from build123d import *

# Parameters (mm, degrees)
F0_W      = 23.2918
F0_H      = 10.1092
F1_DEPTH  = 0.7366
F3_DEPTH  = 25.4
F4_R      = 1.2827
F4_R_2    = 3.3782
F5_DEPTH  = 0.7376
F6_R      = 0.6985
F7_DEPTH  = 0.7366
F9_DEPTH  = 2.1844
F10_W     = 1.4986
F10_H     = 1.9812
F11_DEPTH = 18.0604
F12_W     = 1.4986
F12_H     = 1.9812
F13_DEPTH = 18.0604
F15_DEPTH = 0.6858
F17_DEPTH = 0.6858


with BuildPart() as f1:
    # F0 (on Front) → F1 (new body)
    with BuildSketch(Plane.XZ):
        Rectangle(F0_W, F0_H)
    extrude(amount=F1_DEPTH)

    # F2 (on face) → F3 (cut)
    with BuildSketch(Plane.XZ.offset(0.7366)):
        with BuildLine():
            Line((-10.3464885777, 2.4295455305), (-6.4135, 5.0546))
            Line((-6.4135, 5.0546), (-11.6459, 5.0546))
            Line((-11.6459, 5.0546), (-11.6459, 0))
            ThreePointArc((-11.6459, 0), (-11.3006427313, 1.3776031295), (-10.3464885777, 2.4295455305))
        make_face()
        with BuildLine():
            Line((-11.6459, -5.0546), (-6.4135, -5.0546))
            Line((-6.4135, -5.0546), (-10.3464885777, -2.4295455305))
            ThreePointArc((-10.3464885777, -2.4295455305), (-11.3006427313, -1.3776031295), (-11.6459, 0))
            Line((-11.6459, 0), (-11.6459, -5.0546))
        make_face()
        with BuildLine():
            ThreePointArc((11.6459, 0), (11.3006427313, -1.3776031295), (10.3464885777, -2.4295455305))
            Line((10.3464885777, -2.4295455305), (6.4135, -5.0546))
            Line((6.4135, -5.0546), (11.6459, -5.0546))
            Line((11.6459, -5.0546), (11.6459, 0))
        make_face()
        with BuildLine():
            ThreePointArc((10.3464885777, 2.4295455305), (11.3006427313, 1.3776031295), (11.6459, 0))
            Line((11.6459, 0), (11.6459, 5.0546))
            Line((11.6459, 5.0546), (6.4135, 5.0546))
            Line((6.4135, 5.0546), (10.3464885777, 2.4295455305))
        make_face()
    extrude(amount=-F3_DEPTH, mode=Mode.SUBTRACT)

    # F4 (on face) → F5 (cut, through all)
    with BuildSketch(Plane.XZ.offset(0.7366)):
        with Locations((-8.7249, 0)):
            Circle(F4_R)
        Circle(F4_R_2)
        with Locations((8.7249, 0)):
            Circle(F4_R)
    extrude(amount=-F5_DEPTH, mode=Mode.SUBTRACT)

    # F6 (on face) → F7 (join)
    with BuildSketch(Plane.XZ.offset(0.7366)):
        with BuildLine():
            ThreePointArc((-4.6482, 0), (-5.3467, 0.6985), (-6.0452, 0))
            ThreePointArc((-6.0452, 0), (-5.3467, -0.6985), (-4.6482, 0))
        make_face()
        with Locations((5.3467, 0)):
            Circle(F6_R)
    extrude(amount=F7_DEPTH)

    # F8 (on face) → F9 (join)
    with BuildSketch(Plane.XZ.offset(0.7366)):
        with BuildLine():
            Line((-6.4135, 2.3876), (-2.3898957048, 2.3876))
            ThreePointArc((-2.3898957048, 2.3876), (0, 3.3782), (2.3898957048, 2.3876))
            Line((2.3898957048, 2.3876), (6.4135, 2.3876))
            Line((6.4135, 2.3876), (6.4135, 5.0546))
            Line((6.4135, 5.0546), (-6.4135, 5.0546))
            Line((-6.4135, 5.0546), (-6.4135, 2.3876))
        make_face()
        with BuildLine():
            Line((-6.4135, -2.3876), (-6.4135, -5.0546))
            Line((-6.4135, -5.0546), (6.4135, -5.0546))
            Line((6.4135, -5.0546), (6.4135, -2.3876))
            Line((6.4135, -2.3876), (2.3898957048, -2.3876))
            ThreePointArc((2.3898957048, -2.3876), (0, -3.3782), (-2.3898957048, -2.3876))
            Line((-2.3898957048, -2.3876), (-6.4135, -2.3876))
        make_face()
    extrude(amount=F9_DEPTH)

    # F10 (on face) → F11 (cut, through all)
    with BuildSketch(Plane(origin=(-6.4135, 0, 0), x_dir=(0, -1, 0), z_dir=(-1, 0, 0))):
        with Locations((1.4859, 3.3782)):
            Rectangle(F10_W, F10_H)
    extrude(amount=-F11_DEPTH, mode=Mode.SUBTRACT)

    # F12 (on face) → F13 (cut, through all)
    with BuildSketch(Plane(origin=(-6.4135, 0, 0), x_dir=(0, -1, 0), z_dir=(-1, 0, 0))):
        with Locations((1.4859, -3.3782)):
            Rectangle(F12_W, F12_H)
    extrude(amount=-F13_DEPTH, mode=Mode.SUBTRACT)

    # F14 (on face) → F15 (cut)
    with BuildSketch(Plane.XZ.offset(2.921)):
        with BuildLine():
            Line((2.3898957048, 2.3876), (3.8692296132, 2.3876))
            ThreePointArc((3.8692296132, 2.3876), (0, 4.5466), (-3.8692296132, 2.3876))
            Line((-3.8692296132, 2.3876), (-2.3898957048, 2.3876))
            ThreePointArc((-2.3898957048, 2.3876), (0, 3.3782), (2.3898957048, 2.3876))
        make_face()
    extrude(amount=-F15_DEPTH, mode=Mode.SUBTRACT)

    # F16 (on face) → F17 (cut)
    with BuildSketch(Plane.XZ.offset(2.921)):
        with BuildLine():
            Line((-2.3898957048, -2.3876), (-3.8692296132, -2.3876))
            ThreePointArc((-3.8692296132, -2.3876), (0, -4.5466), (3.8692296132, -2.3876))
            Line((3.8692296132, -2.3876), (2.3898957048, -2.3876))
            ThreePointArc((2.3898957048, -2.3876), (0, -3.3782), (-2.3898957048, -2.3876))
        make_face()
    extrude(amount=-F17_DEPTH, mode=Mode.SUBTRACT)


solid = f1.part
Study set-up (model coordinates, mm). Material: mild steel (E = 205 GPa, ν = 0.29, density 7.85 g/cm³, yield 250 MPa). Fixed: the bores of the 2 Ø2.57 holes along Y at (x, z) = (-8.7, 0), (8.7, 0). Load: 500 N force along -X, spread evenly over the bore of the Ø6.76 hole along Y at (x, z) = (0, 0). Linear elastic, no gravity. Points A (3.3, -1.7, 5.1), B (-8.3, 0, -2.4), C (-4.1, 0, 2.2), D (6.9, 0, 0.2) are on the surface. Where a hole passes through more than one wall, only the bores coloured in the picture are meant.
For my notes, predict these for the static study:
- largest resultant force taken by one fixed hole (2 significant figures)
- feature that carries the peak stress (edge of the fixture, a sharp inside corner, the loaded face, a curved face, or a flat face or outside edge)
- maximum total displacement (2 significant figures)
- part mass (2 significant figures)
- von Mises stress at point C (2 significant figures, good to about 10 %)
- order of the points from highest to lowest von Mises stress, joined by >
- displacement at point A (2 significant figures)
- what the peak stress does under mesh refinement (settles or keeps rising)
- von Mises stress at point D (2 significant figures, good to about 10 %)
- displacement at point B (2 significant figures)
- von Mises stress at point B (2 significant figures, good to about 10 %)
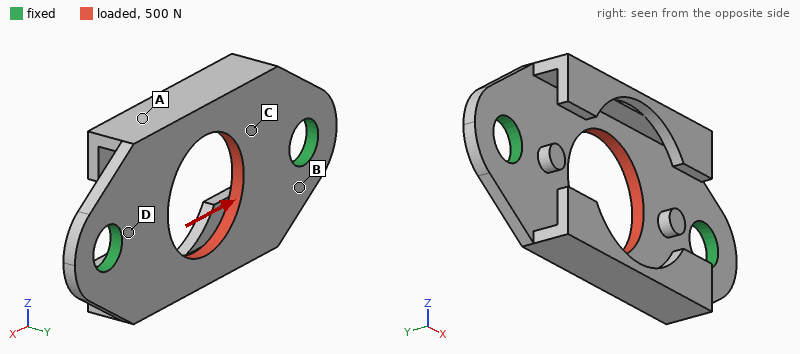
250 N
edge of the fixture
2.1 µm
1.3 g
53 MPa
D > C > B > A
1.4 µm
keeps rising
68 MPa
0.46 µm
31 MPa
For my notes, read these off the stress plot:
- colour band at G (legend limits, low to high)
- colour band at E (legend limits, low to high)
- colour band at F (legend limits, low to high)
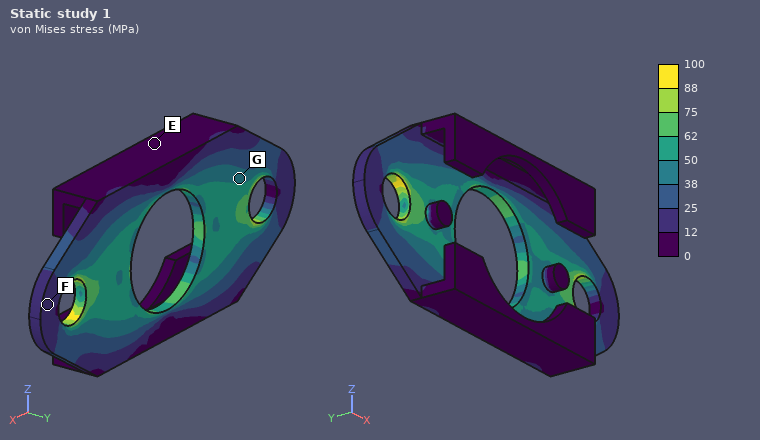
38 to 50 MPa
0 to 12 MPa
12 to 25 MPa
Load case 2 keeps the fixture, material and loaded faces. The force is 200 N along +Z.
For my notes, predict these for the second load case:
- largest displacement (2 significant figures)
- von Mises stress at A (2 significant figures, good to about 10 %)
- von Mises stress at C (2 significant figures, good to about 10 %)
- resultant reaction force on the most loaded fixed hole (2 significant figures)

3.5 µm
7.9 MPa
22 MPa
100 N
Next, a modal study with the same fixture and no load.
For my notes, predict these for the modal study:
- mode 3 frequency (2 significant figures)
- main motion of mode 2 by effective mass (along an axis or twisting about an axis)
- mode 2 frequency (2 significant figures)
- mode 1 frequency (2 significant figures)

24 kHz
along Y
14 kHz
12 kHz
